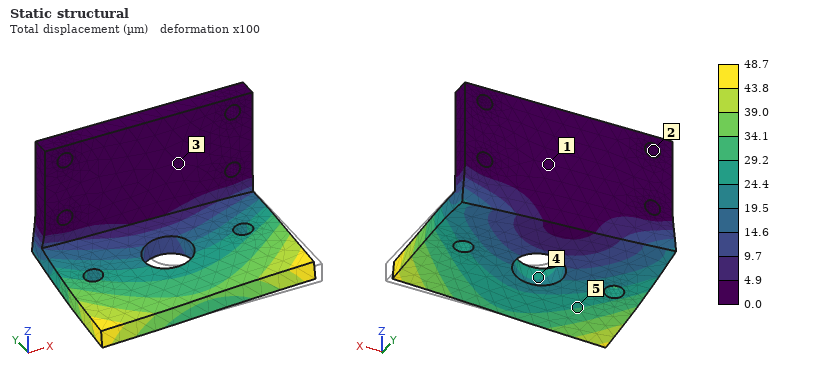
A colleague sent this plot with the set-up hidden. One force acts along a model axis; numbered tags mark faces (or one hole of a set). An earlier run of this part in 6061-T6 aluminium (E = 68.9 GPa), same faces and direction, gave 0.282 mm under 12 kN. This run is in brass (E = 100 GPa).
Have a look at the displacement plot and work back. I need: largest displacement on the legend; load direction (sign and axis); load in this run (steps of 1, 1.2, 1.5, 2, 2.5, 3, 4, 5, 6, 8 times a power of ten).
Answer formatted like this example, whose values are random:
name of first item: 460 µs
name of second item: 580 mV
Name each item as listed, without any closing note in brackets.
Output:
largest displacement on the legend: 48.7 µm
load direction: -X
load in this run: 3 kN
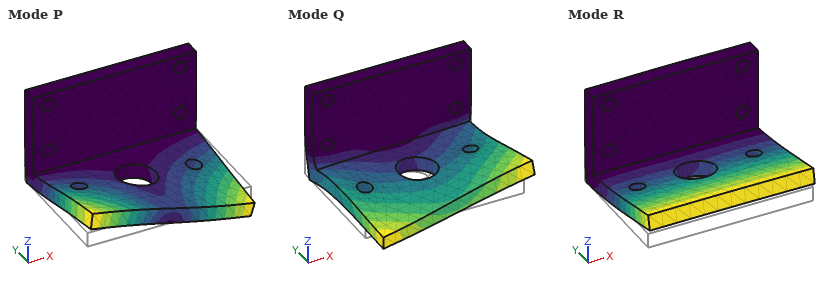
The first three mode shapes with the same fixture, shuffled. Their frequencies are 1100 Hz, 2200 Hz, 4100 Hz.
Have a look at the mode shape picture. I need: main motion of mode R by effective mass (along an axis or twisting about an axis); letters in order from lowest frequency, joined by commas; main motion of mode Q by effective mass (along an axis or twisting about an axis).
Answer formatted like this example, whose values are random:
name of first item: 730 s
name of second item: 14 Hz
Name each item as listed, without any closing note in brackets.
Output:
main motion of mode R by effective mass: along Z
letters in order from lowest frequency, joined by commas: R, P, Q
main motion of mode Q by effective mass: along X
